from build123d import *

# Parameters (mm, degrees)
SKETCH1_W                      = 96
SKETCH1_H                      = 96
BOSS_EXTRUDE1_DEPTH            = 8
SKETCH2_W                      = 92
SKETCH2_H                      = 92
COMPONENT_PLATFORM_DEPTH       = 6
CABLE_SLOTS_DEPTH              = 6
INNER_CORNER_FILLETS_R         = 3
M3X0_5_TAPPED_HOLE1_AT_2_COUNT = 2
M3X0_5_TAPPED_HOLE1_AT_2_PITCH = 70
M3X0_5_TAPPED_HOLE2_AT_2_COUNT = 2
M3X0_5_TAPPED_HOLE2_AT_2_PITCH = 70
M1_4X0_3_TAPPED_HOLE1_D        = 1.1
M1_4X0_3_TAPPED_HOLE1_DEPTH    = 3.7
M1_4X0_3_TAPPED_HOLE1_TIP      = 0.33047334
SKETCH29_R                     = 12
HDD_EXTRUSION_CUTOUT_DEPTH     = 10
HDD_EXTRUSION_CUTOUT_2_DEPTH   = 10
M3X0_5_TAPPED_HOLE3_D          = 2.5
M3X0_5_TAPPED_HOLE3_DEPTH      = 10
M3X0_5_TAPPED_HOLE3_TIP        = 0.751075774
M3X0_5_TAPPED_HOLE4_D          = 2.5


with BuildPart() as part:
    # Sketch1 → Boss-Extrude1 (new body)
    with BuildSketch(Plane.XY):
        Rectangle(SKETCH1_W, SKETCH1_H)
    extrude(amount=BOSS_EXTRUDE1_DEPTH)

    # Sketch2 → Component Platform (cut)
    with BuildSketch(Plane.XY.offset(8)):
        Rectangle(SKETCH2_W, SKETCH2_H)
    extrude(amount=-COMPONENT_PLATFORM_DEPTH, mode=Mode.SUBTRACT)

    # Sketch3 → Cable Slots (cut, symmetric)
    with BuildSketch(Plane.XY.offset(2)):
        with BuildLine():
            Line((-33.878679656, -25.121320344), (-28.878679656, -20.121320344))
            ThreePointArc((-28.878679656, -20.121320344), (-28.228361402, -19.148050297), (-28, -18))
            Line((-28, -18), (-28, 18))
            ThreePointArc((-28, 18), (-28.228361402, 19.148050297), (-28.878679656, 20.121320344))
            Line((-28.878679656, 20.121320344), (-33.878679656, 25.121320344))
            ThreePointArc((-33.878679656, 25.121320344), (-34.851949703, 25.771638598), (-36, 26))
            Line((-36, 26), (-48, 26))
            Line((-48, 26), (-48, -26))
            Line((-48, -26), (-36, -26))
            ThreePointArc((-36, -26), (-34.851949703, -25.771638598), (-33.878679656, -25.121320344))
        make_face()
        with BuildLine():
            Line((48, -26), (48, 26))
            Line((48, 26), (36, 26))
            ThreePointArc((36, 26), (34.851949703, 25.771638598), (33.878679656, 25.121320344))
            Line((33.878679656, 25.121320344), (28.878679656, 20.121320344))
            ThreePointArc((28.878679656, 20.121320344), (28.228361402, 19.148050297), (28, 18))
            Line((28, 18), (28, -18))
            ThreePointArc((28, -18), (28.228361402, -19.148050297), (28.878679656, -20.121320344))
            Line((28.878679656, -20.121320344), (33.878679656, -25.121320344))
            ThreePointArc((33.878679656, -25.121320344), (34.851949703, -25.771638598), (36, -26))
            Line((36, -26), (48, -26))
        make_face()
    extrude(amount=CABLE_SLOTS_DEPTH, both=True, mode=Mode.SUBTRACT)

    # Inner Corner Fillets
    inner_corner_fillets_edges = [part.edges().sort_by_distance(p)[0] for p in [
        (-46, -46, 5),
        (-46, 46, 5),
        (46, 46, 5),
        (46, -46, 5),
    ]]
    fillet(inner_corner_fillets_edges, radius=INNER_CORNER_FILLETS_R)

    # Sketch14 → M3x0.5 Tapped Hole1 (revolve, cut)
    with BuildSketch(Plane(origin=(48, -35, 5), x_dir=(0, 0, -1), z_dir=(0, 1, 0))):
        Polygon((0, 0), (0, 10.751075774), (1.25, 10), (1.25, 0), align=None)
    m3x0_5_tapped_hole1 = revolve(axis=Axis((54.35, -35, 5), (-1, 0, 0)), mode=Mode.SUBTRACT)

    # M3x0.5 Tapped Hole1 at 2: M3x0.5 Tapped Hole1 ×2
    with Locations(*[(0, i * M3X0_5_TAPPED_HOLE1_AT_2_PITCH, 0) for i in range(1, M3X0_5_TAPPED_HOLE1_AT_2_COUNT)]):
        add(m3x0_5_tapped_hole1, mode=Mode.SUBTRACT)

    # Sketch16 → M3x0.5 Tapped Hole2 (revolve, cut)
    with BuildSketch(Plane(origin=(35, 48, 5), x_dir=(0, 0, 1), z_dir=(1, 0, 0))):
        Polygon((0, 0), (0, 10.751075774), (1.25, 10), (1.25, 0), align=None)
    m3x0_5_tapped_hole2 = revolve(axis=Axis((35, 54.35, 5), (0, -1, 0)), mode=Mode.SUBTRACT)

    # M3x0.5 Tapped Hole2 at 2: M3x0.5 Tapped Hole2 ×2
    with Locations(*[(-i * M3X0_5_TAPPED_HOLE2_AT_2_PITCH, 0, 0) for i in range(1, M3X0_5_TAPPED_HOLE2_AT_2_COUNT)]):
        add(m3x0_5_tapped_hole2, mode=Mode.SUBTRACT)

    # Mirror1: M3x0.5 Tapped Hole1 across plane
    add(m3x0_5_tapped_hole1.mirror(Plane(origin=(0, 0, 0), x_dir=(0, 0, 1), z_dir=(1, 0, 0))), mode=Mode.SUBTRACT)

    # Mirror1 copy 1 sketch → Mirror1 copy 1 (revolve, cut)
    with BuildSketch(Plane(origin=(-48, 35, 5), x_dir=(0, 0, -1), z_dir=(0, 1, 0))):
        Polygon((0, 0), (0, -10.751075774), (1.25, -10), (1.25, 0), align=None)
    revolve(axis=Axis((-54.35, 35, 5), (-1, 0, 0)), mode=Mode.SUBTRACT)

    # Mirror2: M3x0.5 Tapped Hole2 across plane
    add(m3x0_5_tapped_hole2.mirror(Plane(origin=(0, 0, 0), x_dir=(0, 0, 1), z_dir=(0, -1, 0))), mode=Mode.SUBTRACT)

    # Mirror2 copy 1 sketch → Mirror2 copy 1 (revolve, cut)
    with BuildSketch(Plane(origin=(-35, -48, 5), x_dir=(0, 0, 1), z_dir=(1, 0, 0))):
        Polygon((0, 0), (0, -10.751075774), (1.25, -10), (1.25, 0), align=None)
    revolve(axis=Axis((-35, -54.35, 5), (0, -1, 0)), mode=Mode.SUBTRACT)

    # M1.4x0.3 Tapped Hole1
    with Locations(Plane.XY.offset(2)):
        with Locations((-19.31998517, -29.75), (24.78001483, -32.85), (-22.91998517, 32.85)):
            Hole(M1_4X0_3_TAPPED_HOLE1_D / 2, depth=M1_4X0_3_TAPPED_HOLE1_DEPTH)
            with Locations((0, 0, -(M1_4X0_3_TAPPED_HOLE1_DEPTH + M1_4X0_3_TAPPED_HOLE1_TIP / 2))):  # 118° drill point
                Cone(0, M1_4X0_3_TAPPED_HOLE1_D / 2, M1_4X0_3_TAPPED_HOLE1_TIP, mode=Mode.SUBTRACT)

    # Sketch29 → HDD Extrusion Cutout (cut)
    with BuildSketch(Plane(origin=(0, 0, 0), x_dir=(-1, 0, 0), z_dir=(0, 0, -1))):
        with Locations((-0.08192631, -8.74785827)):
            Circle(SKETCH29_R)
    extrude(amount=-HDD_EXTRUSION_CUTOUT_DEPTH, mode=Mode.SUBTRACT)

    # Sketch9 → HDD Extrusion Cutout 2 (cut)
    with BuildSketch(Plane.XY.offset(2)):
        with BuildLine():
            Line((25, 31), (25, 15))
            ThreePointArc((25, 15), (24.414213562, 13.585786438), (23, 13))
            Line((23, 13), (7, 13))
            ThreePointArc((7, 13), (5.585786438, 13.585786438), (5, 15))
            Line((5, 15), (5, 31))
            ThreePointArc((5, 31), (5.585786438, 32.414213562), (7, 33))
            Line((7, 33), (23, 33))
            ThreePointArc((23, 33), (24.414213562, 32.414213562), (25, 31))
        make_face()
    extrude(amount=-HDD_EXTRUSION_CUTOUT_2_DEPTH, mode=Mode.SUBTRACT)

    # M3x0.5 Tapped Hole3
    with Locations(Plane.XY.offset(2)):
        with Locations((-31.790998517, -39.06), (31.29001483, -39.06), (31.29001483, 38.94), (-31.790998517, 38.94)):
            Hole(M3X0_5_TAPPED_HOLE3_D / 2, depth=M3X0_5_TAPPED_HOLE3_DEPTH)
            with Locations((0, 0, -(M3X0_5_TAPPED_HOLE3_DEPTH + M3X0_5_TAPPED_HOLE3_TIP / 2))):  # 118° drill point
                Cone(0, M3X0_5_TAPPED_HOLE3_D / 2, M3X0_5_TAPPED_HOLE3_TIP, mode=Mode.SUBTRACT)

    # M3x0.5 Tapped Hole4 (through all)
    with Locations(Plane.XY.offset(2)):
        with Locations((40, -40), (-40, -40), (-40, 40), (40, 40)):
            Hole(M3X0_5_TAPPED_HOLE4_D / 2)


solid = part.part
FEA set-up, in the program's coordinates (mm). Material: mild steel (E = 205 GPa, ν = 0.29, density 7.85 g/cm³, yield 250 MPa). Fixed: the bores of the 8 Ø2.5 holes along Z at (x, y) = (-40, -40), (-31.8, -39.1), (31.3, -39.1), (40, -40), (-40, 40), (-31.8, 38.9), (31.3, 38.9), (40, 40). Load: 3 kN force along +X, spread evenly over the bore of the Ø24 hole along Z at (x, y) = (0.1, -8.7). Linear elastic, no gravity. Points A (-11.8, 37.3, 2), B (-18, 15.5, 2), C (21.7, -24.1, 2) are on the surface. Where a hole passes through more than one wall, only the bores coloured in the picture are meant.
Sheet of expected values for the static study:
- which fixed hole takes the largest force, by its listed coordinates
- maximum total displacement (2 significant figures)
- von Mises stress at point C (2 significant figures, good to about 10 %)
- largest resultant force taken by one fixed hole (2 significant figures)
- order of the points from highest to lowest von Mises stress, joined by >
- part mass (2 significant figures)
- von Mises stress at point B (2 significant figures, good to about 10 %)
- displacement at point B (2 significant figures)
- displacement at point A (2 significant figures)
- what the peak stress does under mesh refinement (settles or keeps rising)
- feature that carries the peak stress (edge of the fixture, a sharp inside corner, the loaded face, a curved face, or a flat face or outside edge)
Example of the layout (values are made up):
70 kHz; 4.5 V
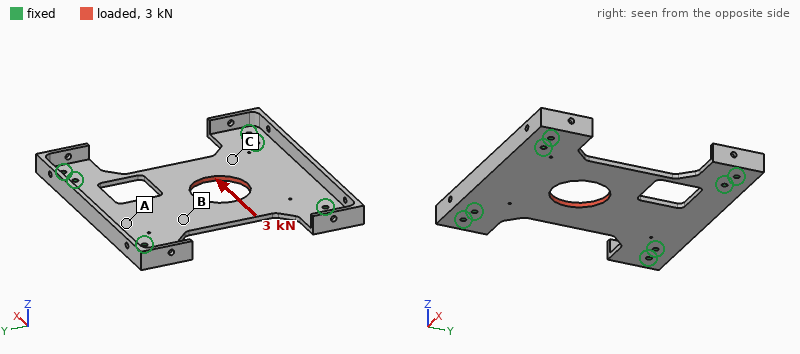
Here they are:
(-31.8, -39.1); 11 µm; 20 MPa; 770 N; B > C > A; 120 g; 28 MPa; 6.7 µm; 2.4 µm; keeps rising; a sharp inside corner
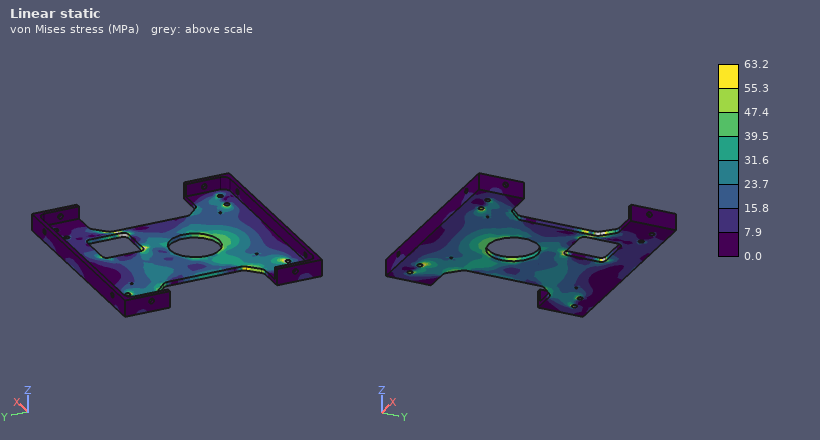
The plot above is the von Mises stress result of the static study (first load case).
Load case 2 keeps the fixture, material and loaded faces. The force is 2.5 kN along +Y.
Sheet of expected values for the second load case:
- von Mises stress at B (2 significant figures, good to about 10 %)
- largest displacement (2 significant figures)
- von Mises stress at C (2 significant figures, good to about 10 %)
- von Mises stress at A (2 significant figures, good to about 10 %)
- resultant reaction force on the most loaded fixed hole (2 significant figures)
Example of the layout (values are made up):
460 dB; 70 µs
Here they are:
12 MPa; 8.3 µm; 18 MPa; 6.3 MPa; 820 N
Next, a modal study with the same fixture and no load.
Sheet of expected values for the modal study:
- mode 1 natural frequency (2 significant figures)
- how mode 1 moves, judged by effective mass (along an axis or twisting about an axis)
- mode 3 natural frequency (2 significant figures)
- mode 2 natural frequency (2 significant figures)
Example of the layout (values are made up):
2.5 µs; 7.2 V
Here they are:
1400 Hz; along Z; 3200 Hz; 2500 Hz
